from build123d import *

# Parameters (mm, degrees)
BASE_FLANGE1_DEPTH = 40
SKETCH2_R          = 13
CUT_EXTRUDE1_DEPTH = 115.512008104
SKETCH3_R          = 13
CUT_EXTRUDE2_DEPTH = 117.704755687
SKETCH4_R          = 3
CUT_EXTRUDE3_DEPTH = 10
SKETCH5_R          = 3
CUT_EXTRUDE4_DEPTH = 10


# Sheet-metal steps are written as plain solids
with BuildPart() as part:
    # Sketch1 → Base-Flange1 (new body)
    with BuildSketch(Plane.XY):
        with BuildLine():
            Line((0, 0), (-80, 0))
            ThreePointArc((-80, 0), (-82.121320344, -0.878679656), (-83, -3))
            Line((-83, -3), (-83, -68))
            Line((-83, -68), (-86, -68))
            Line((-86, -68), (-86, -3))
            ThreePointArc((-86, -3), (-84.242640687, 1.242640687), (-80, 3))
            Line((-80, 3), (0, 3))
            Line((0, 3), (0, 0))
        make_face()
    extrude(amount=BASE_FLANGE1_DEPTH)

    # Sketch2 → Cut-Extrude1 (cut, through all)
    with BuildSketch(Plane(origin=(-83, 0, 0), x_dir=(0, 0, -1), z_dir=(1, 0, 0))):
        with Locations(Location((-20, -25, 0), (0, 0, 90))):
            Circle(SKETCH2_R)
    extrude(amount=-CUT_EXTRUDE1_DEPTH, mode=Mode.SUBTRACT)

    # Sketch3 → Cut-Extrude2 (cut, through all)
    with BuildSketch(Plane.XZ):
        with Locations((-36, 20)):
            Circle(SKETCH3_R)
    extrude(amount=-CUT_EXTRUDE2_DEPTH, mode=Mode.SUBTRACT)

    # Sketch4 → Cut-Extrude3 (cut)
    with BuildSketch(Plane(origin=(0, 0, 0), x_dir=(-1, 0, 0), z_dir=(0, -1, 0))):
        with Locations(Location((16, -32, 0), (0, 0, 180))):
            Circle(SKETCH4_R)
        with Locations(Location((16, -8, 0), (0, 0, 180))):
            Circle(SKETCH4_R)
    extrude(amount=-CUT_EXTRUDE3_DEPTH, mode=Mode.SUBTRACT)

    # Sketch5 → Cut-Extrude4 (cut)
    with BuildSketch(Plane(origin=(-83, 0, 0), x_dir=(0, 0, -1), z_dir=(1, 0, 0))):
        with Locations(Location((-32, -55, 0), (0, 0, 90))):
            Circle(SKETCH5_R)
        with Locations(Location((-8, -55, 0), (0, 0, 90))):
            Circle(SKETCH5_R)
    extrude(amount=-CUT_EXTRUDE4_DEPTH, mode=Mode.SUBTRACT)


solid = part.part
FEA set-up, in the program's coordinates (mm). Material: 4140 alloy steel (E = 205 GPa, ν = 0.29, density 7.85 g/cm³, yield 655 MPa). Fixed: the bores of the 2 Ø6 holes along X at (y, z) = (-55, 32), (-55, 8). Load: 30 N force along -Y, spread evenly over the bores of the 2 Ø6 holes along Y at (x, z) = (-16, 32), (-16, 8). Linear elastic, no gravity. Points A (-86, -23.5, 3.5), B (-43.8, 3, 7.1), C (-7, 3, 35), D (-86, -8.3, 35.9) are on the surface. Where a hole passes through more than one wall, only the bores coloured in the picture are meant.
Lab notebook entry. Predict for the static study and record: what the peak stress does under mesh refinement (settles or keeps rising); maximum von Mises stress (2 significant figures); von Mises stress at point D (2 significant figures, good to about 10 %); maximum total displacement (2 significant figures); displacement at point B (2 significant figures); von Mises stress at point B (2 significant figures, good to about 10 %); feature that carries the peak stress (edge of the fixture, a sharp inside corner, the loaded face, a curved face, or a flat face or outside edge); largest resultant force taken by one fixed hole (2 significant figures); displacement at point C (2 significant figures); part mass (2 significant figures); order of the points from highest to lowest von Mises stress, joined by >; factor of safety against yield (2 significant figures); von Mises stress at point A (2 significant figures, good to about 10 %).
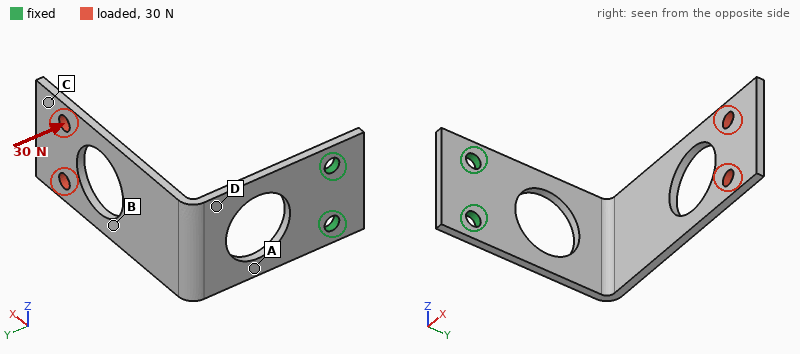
settles
110 MPa
43 MPa
1.2 mm
0.57 mm
33 MPa
a curved face
15 N
1.1 mm
120 g
A > D > B > C
5.7
94 MPa
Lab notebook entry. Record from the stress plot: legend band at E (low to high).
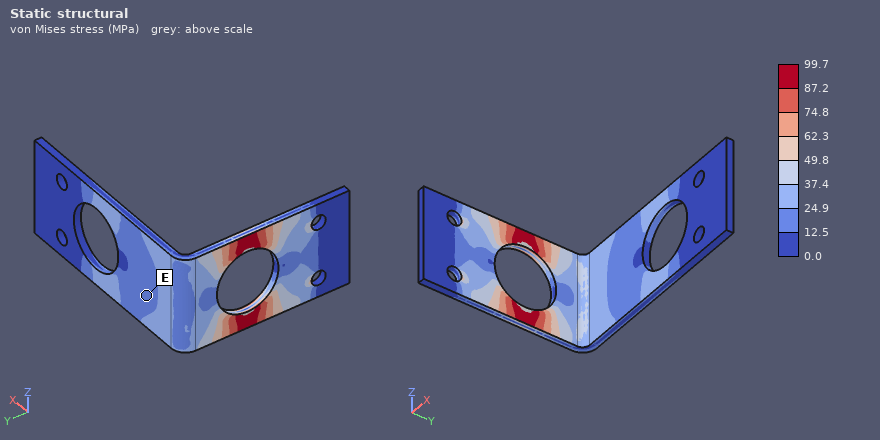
12.5 to 24.9 MPa
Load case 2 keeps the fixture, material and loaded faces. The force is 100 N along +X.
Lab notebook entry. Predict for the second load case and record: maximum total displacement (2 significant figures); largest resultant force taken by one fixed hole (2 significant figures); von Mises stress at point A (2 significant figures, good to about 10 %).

1.3 mm
50 N
120 MPa
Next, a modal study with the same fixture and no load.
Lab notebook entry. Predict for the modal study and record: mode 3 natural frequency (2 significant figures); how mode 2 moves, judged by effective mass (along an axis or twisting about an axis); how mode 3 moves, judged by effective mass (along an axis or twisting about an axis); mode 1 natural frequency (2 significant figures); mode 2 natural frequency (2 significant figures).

500 Hz
along Z
along X
150 Hz
260 Hz
